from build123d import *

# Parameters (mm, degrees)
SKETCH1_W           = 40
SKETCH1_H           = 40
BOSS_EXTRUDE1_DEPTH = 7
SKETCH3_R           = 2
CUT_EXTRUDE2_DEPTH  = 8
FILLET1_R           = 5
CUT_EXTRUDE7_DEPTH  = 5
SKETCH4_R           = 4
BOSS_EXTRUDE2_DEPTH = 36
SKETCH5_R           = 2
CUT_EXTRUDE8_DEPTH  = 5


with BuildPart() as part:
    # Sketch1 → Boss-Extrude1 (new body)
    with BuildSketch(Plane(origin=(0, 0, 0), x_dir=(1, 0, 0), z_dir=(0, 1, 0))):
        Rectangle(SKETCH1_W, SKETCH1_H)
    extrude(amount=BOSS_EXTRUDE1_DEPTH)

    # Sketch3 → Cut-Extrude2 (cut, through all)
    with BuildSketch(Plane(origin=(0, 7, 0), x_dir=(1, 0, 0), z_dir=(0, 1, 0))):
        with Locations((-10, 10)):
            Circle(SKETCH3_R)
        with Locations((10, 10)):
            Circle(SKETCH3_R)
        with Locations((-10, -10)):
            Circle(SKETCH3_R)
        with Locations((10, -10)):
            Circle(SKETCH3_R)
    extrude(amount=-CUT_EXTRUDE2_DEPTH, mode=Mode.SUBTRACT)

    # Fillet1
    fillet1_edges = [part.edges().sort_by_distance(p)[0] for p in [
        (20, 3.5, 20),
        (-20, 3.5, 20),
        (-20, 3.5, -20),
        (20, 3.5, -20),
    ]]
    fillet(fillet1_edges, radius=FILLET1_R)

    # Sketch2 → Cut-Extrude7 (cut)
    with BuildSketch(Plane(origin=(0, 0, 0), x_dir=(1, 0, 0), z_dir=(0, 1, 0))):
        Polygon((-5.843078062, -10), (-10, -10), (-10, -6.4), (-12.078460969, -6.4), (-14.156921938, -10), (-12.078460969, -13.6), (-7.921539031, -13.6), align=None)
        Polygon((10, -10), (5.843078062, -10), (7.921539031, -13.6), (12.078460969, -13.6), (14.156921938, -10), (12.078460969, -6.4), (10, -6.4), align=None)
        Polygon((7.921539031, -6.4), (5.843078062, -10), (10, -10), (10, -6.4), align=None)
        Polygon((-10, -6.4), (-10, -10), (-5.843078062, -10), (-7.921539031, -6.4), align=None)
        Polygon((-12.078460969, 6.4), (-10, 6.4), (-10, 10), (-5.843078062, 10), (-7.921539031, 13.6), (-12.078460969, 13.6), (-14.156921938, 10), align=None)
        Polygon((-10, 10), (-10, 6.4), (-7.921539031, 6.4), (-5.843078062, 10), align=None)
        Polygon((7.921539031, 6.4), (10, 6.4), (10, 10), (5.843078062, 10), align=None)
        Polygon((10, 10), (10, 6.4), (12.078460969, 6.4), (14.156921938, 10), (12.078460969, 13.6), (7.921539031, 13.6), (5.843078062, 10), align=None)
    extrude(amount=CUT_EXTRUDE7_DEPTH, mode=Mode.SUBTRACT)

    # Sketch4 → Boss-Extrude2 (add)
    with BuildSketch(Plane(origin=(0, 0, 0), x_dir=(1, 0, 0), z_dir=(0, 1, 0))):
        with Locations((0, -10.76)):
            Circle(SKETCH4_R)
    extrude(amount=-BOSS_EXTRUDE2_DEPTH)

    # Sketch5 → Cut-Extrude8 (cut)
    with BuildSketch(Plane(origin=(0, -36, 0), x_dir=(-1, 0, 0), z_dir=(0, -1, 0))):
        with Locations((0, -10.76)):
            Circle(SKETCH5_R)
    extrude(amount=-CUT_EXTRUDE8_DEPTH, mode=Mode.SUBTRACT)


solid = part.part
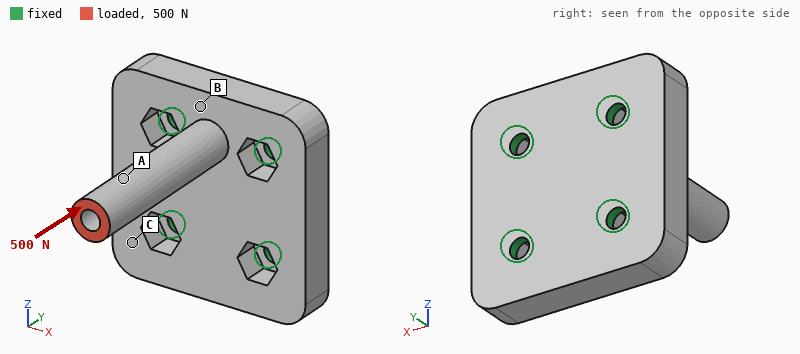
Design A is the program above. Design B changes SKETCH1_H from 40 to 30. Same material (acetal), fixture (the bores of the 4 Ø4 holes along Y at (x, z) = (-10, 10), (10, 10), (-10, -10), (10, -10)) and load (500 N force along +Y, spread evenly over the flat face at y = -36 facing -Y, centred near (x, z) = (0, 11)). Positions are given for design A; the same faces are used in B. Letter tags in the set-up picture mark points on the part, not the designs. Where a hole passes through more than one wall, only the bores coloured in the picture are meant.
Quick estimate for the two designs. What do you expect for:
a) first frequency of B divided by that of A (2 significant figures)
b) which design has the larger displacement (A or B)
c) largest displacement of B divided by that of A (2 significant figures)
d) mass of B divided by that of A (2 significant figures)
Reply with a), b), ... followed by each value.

a) 0.97
b) B
c) 1.3
d) 0.76
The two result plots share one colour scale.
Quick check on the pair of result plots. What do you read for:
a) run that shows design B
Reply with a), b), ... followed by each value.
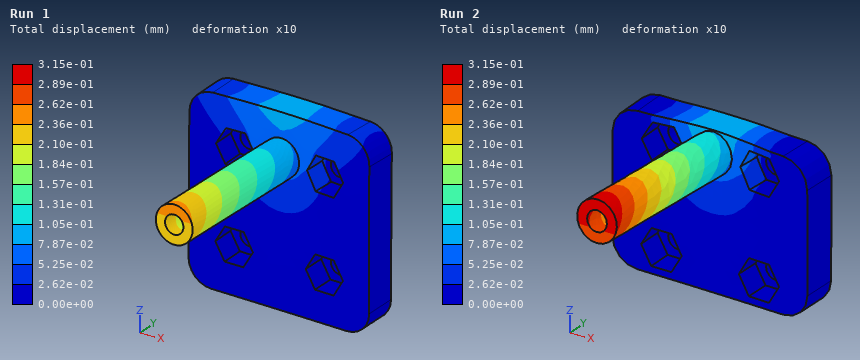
a) Run 2
